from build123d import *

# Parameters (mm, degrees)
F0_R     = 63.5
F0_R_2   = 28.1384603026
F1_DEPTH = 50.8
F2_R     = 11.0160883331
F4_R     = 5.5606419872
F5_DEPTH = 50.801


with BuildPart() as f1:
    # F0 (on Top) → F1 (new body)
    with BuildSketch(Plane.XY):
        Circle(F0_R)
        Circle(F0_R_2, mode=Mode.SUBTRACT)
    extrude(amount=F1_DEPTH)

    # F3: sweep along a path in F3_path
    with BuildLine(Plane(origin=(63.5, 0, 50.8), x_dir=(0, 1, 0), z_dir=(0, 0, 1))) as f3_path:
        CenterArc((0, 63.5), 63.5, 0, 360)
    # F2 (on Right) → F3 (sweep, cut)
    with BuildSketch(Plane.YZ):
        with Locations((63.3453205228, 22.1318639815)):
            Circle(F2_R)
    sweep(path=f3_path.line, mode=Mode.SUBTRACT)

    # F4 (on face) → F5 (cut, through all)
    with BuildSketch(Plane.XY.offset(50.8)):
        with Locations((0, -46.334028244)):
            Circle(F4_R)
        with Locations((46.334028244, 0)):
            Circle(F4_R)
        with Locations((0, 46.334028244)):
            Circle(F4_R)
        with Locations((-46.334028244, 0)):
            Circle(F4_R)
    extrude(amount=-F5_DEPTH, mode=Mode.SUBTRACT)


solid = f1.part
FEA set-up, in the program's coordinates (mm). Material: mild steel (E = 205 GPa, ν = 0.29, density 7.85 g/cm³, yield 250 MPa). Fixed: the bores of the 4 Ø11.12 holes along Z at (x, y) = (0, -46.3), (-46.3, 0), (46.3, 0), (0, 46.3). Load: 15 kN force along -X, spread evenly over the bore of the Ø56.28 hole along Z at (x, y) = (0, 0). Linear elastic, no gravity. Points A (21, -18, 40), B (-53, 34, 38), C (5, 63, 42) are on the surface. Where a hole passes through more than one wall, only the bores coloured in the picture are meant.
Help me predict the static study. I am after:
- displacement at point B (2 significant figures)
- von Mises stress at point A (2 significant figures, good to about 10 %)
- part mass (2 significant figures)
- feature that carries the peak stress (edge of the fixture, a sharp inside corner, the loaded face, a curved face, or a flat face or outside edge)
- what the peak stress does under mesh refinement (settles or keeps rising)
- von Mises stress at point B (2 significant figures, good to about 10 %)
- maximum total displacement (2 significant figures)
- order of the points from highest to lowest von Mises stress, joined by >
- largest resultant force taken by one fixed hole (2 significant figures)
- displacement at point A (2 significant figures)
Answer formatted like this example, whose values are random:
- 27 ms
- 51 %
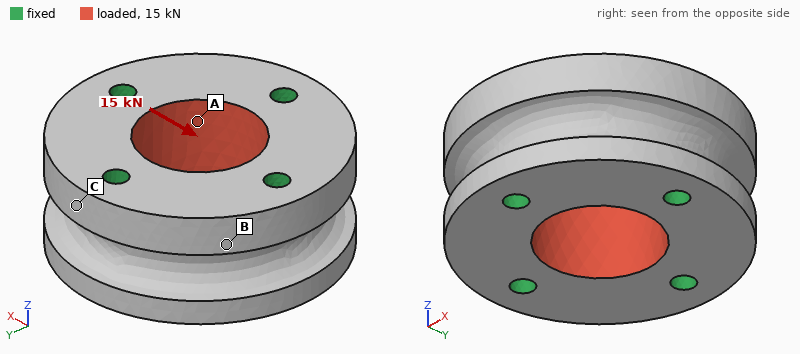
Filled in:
- 0.24 µm
- 2.1 MPa
- 3.3 kg
- edge of the fixture
- keeps rising
- 1.1 MPa
- 0.44 µm
- A > B > C
- 3.8 kN
- 0.39 µm
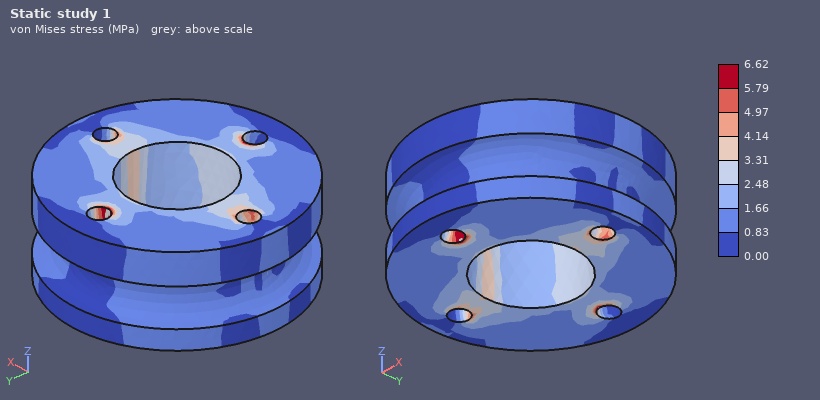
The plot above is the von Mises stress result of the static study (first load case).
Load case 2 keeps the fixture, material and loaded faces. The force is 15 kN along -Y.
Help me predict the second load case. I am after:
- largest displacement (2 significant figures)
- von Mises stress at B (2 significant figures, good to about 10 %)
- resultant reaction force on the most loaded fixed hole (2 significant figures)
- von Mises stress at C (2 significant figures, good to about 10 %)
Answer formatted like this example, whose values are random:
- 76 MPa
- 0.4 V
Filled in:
- 0.44 µm
- 1.1 MPa
- 3.8 kN
- 1.0 MPa
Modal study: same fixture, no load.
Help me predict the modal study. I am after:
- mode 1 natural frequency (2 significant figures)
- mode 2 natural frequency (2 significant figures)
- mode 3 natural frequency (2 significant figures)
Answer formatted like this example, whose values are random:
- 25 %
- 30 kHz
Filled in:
- 16 kHz
- 17 kHz
- 17 kHz
